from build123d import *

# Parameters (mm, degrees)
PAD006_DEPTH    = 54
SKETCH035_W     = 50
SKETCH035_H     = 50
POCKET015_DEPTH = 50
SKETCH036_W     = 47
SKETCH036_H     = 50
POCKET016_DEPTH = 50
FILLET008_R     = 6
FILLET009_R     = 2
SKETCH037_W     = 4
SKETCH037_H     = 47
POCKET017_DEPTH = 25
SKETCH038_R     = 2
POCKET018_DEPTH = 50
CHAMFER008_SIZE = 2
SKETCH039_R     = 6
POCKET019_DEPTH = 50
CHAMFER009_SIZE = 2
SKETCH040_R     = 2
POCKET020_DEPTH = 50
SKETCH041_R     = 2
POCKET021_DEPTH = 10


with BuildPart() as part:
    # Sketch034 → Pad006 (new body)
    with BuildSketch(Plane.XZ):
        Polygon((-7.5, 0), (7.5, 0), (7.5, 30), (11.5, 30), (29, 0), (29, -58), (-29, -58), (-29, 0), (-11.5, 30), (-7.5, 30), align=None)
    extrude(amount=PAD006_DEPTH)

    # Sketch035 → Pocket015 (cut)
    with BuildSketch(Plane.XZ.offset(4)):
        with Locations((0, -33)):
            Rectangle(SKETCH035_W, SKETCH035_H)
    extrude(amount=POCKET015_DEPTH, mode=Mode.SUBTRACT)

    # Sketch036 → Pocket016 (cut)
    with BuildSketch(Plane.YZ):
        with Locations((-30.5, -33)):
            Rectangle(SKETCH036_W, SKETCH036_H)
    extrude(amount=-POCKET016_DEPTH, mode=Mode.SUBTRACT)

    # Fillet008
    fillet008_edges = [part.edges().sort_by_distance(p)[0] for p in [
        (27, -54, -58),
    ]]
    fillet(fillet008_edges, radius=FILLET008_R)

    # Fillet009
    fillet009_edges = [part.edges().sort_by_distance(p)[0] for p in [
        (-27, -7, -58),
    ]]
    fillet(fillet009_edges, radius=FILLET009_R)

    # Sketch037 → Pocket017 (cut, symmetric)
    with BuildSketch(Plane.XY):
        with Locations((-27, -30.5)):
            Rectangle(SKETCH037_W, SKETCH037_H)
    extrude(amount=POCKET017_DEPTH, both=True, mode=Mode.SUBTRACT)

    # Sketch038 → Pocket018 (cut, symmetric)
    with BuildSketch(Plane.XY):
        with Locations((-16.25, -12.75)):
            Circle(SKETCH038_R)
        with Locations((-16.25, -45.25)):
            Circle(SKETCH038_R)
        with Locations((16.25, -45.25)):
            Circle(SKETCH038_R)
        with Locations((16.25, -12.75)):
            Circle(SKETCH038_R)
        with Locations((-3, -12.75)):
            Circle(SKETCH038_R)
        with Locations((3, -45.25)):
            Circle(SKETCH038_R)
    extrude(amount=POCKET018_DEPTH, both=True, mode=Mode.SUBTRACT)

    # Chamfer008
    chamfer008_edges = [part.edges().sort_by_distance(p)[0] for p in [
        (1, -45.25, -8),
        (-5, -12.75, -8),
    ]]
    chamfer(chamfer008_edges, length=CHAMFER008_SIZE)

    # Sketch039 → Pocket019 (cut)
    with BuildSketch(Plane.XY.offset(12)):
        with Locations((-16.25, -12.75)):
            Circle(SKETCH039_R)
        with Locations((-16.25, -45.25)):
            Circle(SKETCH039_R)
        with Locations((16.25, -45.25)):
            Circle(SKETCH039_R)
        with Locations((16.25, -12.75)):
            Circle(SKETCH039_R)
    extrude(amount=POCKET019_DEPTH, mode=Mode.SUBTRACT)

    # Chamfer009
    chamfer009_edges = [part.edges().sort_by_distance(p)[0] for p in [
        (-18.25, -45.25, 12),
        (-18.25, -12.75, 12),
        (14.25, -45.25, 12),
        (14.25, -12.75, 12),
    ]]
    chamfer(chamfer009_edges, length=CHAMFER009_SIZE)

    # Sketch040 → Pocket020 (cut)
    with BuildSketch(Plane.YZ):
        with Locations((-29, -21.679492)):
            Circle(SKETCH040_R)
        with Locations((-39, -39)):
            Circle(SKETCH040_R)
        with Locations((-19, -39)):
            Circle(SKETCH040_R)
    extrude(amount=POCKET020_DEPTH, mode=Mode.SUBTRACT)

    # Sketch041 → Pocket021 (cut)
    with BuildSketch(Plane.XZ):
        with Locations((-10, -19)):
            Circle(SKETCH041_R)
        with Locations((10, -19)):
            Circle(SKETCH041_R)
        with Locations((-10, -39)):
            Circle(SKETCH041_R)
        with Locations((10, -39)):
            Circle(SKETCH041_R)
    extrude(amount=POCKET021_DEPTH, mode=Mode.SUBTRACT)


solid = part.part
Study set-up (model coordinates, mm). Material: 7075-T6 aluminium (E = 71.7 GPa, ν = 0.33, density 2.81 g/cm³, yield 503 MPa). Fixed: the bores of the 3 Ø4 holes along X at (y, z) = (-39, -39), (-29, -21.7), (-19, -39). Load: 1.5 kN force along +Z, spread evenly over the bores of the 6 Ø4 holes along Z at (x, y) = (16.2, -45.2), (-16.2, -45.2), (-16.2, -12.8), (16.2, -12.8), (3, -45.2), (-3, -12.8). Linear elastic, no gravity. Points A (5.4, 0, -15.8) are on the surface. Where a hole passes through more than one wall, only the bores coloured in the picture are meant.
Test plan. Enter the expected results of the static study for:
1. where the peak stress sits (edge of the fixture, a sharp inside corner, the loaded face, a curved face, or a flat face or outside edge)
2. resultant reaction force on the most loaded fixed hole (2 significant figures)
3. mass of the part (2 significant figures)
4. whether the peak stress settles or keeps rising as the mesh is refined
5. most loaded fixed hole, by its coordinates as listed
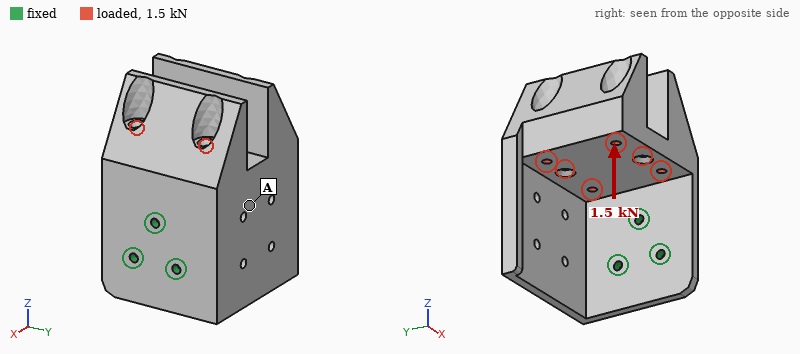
edge of the fixture
1.5 kN
230 g
keeps rising
(-29, -21.7)
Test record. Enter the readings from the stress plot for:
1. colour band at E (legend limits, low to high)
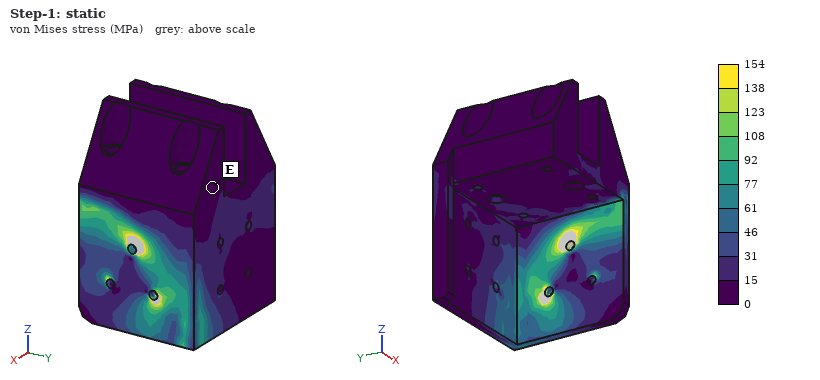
0 to 15 MPa
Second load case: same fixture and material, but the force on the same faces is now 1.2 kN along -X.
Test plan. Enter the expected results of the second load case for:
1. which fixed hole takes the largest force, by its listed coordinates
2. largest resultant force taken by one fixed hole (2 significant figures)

(-29, -21.7)
1.9 kN
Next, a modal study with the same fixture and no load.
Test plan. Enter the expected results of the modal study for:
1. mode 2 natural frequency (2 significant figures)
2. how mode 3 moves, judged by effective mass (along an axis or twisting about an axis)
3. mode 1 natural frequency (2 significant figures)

850 Hz
along X
490 Hz
